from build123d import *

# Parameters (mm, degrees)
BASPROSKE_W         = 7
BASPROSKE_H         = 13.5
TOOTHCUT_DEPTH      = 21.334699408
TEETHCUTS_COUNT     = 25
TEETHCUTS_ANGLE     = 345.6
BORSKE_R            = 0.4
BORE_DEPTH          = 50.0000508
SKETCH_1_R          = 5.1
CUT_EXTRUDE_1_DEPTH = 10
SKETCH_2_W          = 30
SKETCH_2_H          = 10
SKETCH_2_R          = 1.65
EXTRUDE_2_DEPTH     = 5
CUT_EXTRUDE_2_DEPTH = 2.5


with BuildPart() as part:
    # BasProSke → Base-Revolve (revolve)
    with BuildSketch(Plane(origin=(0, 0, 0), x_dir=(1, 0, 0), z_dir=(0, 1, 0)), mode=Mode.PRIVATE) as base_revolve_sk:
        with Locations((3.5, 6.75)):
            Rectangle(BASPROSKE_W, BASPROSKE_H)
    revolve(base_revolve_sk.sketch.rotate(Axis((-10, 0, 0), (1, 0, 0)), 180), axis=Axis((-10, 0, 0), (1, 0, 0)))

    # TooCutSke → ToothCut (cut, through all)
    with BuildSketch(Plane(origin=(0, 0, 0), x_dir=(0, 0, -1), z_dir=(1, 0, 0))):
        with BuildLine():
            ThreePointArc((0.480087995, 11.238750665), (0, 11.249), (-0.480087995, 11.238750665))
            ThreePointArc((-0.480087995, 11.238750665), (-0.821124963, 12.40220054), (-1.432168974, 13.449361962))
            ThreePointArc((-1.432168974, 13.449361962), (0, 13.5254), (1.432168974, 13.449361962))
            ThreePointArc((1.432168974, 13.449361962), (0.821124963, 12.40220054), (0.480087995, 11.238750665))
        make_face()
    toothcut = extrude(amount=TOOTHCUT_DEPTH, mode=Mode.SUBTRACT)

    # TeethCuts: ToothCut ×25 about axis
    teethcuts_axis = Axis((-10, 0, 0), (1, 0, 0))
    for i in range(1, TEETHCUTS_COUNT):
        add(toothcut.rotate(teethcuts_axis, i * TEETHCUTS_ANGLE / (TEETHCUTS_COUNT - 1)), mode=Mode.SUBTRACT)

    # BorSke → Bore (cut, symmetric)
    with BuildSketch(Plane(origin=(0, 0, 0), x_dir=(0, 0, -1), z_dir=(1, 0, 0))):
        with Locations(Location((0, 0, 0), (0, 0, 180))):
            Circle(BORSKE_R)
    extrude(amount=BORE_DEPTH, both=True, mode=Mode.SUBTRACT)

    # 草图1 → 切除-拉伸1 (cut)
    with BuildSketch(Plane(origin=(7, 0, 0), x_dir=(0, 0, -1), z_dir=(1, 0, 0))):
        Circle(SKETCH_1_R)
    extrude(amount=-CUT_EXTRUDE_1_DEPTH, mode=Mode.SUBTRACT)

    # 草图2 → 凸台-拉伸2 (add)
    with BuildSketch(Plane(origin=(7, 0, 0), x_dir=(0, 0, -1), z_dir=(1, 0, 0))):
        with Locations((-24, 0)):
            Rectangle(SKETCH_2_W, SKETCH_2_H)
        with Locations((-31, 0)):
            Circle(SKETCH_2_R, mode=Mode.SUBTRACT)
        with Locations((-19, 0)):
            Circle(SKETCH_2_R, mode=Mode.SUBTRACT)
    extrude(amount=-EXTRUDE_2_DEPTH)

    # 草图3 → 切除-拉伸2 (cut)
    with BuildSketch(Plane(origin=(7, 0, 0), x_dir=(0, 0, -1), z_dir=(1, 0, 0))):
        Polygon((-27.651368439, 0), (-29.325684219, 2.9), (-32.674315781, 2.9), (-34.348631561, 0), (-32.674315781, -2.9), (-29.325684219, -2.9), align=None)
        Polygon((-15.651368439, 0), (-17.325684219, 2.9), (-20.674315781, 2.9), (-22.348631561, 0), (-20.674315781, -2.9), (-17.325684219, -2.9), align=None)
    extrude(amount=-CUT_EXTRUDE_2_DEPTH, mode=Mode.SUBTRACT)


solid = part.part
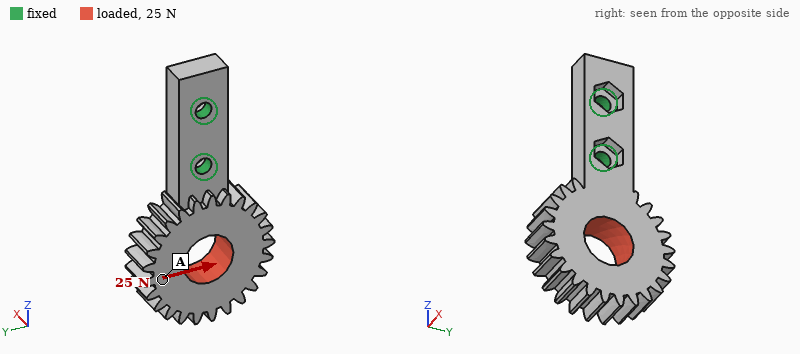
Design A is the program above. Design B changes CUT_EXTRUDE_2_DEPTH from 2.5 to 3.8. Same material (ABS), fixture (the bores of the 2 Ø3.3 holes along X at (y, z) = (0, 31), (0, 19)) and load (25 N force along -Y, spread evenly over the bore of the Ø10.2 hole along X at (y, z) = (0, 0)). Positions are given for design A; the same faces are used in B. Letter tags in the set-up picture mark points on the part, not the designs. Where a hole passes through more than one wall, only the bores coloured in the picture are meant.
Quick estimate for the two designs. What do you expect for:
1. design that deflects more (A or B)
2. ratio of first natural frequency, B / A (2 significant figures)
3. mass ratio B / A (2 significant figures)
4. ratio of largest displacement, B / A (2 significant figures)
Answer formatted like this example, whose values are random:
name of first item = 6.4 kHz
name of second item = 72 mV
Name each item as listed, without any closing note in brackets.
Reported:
design that deflects more = B
ratio of first natural frequency, B / A = 0.92
mass ratio B / A = 0.99
ratio of largest displacement, B / A = 1.2
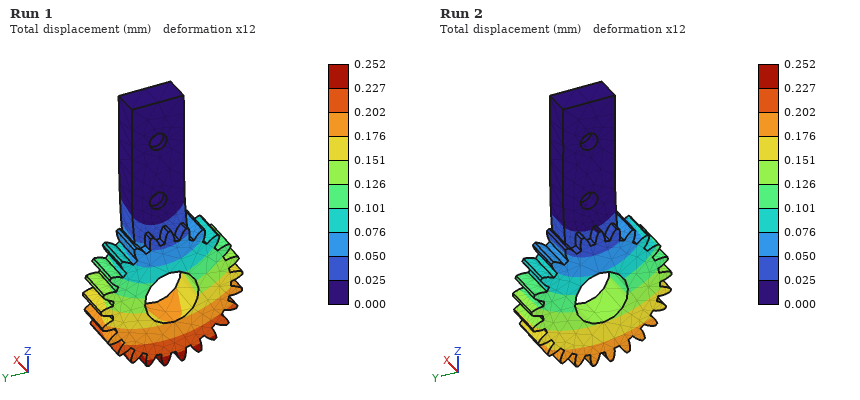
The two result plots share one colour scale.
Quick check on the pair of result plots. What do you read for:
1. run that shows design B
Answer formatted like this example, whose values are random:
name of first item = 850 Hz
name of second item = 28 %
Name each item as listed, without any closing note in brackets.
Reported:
run that shows design B = Run 1
